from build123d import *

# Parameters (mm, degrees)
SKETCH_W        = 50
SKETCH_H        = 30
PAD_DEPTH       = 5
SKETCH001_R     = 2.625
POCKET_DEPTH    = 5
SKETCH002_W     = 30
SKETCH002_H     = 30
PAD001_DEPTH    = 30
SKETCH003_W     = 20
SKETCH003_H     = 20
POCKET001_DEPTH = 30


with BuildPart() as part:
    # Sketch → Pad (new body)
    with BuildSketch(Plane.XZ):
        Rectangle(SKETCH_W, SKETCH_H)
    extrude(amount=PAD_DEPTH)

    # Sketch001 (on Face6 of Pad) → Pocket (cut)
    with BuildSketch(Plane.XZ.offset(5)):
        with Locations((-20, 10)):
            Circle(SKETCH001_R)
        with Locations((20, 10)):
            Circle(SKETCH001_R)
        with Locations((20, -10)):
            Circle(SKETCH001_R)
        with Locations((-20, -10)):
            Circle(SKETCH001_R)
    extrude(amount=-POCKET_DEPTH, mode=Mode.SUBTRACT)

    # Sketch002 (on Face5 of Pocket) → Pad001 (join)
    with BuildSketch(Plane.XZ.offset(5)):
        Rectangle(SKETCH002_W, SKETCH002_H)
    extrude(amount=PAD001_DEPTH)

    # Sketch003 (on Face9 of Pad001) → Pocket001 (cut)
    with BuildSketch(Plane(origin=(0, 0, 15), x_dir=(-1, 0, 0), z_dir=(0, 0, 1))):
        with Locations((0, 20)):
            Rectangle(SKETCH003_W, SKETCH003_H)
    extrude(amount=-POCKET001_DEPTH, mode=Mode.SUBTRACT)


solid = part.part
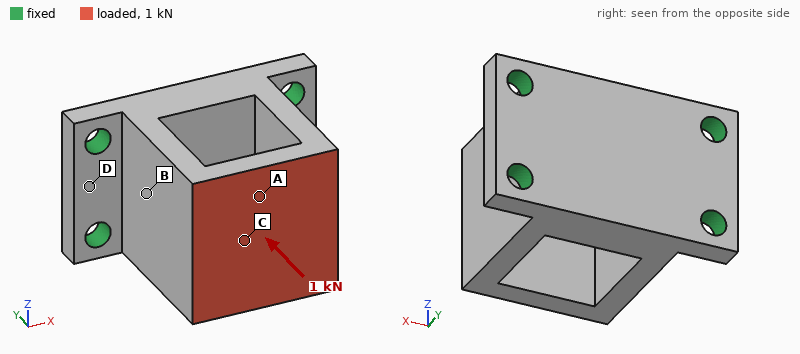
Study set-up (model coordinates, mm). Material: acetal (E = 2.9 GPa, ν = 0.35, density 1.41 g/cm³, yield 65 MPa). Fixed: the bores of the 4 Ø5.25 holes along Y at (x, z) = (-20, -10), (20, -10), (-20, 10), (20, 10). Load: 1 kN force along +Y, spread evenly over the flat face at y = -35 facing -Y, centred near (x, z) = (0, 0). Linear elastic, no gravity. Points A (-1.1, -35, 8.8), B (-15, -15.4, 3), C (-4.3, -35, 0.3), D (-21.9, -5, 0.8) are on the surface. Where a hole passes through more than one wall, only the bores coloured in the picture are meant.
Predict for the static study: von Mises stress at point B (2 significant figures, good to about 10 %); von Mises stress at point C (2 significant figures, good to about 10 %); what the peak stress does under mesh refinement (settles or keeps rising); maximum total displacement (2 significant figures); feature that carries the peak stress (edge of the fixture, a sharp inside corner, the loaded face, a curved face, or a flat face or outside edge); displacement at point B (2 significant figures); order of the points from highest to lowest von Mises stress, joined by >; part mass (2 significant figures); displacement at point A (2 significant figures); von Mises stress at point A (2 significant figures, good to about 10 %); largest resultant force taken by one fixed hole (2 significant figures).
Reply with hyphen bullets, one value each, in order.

- 3.3 MPa
- 6.4 MPa
- keeps rising
- 0.15 mm
- edge of the fixture
- 0.052 mm
- A > C > B > D
- 31 g
- 0.14 mm
- 9.0 MPa
- 260 N
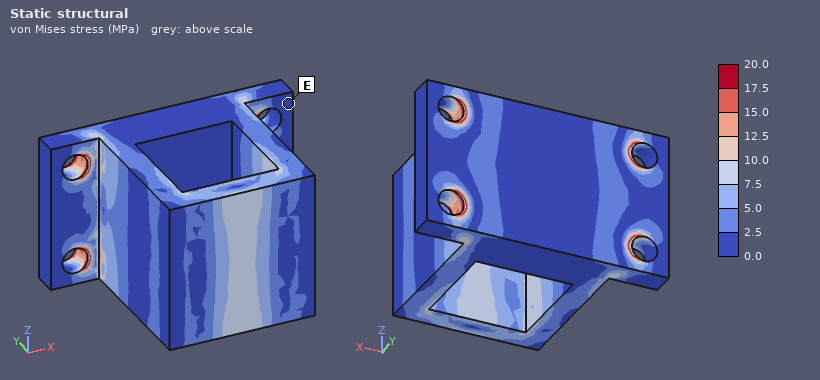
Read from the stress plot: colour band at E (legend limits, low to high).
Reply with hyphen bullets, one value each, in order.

- 0.0 to 2.5 MPa
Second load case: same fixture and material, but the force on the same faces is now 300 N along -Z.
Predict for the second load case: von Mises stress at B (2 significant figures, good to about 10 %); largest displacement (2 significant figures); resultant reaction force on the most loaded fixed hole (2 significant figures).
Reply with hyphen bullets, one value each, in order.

- 2.4 MPa
- 0.21 mm
- 250 N
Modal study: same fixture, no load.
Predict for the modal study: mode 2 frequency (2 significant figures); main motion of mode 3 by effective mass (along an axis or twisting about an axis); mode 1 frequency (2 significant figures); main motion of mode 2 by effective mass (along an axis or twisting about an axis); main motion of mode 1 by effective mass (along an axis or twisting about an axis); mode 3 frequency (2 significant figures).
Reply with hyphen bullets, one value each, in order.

- 2100 Hz
- twisting about Y
- 1600 Hz
- along Z
- along X
- 3300 Hz
